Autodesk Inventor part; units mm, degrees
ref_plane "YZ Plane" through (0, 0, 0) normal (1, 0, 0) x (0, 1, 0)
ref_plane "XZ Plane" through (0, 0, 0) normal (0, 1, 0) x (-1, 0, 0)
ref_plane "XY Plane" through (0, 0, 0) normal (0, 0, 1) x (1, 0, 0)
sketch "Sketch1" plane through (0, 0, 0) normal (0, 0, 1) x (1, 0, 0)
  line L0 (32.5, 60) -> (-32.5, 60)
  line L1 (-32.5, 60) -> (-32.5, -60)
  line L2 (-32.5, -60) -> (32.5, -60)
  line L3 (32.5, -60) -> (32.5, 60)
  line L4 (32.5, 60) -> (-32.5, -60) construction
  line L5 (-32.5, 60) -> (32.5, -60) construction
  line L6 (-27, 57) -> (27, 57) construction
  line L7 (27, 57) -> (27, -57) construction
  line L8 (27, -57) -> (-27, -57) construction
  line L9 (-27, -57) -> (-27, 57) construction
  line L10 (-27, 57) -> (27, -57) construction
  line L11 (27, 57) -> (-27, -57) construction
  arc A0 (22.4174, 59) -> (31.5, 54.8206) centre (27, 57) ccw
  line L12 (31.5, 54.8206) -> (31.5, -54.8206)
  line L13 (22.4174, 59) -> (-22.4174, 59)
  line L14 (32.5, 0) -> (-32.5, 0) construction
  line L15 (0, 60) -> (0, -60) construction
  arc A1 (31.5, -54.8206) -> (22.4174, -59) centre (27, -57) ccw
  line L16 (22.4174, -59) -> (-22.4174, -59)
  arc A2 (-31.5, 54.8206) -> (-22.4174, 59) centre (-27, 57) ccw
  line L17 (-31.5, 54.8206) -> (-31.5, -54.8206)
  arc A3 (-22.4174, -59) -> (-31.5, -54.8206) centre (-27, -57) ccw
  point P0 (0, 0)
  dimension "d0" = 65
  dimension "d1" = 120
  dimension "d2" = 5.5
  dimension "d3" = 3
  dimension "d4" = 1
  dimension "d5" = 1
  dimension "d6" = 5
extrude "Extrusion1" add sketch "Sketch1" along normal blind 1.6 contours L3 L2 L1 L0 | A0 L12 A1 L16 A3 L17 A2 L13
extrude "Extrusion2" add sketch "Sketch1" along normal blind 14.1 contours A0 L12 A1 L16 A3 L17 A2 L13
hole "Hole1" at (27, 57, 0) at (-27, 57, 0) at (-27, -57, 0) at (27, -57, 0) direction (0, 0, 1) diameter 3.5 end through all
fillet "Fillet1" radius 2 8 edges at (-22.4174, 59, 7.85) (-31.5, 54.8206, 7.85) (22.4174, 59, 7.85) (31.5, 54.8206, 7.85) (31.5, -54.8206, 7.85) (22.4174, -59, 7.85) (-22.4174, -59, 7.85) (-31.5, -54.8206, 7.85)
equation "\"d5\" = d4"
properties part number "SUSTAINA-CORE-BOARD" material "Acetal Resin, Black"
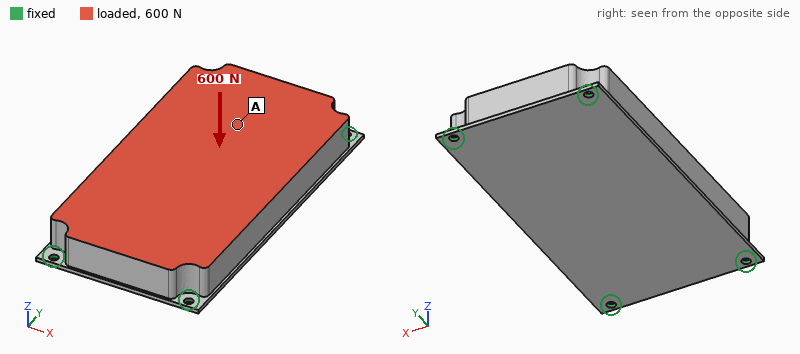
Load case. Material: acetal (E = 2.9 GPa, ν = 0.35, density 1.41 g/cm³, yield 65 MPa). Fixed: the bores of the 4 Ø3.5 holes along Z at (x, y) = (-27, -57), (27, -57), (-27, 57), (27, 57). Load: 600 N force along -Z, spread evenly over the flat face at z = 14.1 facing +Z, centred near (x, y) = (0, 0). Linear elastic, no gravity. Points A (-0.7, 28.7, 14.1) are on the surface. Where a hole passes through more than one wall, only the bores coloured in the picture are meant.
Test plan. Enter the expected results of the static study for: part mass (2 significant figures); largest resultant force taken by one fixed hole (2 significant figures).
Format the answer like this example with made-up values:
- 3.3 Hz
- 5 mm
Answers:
- 140 g
- 230 N
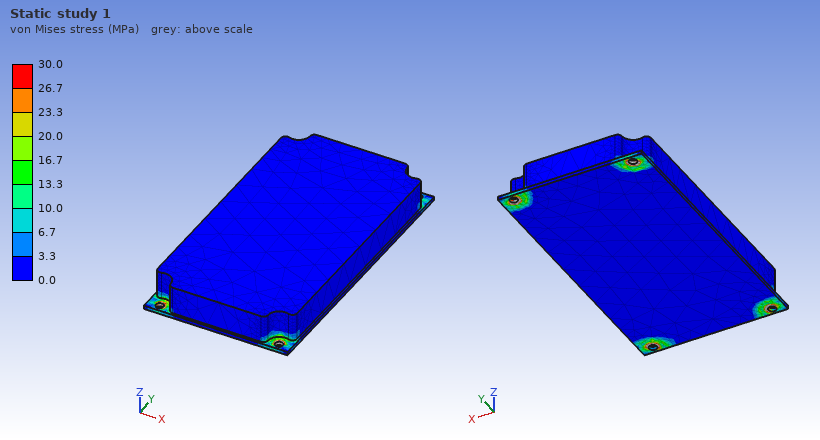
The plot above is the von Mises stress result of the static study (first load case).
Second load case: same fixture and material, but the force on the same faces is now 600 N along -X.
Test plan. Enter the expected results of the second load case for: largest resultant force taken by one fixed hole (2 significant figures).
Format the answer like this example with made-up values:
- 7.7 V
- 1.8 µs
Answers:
- 190 N
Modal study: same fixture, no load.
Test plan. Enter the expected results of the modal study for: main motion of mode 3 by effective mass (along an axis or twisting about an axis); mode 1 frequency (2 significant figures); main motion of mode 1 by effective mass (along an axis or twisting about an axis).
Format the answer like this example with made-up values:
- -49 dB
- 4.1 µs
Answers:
- twisting about X
- 700 Hz
- along Z
